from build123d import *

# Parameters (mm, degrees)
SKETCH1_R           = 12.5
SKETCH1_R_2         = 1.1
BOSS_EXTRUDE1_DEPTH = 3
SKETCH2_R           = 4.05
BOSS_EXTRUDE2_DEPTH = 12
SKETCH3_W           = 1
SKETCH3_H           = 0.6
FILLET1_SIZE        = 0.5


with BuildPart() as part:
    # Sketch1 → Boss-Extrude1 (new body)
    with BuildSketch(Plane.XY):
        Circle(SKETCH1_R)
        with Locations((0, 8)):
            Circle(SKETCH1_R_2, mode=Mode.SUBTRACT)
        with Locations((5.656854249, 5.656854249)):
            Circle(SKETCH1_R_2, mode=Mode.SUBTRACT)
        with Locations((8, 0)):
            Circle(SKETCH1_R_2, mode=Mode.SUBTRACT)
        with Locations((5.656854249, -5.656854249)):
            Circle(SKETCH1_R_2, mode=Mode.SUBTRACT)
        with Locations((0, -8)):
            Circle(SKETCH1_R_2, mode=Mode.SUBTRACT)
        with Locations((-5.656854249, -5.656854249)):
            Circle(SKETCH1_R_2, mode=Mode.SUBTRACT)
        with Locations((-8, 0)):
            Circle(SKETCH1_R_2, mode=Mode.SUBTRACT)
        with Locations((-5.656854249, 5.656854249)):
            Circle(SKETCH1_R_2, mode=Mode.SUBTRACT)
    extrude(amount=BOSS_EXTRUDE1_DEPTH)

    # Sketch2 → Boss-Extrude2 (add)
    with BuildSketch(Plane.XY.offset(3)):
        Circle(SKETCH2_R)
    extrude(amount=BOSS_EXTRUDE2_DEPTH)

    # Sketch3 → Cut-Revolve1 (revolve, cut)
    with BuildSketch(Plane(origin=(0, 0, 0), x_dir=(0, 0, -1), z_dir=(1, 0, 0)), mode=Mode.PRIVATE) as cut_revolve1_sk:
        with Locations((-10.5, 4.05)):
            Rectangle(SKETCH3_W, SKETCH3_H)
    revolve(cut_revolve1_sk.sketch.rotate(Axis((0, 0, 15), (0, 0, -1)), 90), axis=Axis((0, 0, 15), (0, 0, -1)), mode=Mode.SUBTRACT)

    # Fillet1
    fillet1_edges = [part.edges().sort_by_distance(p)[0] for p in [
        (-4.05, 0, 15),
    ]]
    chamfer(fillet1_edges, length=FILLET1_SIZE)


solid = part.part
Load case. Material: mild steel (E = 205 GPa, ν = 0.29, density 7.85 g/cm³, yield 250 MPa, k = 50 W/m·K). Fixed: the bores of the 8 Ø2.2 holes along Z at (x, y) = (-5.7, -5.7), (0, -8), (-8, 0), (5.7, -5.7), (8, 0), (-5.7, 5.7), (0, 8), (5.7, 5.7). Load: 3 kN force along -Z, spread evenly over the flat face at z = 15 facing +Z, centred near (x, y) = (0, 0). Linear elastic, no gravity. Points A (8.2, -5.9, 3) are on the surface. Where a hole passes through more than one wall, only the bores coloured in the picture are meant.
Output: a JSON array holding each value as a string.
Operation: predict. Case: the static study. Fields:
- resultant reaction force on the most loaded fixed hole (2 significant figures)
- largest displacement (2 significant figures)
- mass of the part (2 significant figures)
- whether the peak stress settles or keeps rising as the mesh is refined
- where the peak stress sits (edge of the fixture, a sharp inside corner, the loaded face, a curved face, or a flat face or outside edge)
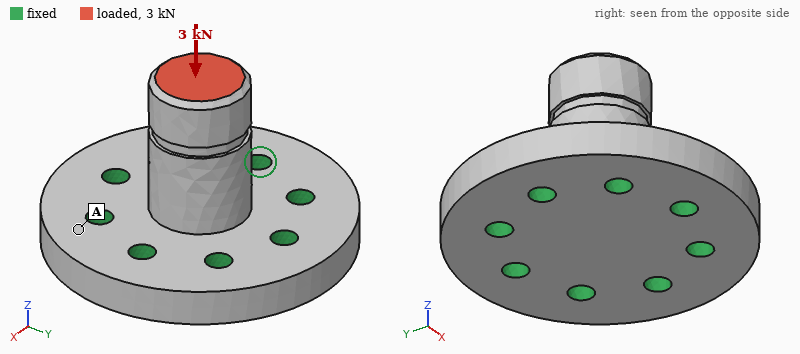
["400 N", "7.0 µm", "16 g", "keeps rising", "edge of the fixture"]
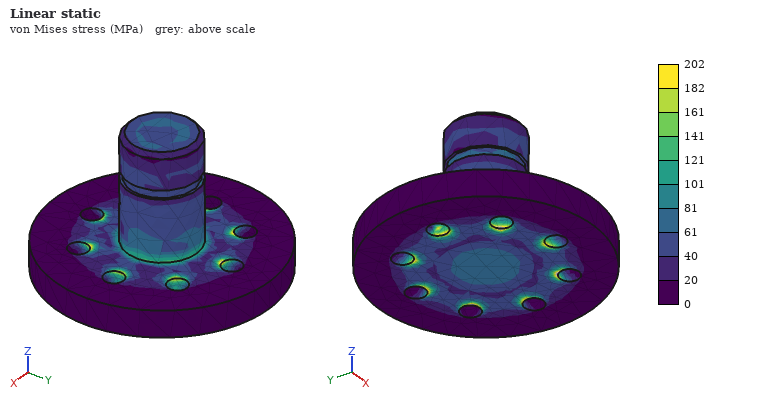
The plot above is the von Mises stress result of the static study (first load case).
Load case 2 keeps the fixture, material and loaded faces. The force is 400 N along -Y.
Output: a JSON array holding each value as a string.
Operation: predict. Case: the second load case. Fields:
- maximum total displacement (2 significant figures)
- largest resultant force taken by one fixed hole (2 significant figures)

["12 µm", "240 N"]
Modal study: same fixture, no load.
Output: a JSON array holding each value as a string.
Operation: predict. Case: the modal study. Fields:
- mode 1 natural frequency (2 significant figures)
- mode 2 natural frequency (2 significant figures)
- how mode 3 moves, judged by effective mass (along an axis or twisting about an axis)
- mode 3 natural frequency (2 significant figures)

["24 kHz", "24 kHz", "along Z", "54 kHz"]
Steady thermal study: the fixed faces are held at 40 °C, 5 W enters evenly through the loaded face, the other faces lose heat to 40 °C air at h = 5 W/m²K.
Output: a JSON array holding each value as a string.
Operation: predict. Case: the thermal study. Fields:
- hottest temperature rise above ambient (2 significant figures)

["30 K"]
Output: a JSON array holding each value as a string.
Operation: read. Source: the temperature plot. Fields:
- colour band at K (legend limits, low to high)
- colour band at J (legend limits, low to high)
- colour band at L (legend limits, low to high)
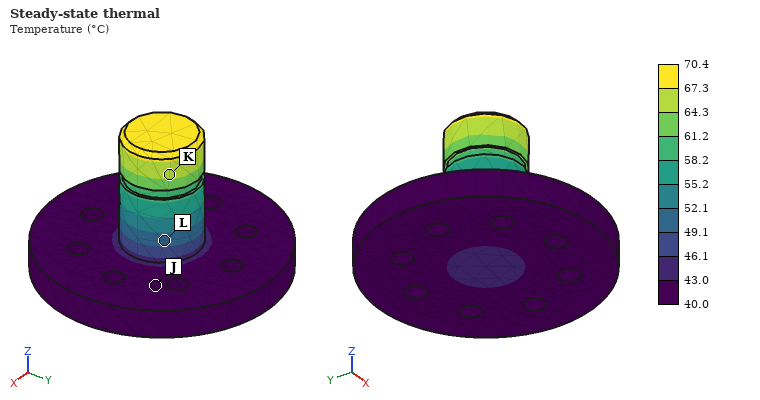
["64.3 to 67.3 °C", "40.0 to 43.0 °C", "49.1 to 52.1 °C"]
